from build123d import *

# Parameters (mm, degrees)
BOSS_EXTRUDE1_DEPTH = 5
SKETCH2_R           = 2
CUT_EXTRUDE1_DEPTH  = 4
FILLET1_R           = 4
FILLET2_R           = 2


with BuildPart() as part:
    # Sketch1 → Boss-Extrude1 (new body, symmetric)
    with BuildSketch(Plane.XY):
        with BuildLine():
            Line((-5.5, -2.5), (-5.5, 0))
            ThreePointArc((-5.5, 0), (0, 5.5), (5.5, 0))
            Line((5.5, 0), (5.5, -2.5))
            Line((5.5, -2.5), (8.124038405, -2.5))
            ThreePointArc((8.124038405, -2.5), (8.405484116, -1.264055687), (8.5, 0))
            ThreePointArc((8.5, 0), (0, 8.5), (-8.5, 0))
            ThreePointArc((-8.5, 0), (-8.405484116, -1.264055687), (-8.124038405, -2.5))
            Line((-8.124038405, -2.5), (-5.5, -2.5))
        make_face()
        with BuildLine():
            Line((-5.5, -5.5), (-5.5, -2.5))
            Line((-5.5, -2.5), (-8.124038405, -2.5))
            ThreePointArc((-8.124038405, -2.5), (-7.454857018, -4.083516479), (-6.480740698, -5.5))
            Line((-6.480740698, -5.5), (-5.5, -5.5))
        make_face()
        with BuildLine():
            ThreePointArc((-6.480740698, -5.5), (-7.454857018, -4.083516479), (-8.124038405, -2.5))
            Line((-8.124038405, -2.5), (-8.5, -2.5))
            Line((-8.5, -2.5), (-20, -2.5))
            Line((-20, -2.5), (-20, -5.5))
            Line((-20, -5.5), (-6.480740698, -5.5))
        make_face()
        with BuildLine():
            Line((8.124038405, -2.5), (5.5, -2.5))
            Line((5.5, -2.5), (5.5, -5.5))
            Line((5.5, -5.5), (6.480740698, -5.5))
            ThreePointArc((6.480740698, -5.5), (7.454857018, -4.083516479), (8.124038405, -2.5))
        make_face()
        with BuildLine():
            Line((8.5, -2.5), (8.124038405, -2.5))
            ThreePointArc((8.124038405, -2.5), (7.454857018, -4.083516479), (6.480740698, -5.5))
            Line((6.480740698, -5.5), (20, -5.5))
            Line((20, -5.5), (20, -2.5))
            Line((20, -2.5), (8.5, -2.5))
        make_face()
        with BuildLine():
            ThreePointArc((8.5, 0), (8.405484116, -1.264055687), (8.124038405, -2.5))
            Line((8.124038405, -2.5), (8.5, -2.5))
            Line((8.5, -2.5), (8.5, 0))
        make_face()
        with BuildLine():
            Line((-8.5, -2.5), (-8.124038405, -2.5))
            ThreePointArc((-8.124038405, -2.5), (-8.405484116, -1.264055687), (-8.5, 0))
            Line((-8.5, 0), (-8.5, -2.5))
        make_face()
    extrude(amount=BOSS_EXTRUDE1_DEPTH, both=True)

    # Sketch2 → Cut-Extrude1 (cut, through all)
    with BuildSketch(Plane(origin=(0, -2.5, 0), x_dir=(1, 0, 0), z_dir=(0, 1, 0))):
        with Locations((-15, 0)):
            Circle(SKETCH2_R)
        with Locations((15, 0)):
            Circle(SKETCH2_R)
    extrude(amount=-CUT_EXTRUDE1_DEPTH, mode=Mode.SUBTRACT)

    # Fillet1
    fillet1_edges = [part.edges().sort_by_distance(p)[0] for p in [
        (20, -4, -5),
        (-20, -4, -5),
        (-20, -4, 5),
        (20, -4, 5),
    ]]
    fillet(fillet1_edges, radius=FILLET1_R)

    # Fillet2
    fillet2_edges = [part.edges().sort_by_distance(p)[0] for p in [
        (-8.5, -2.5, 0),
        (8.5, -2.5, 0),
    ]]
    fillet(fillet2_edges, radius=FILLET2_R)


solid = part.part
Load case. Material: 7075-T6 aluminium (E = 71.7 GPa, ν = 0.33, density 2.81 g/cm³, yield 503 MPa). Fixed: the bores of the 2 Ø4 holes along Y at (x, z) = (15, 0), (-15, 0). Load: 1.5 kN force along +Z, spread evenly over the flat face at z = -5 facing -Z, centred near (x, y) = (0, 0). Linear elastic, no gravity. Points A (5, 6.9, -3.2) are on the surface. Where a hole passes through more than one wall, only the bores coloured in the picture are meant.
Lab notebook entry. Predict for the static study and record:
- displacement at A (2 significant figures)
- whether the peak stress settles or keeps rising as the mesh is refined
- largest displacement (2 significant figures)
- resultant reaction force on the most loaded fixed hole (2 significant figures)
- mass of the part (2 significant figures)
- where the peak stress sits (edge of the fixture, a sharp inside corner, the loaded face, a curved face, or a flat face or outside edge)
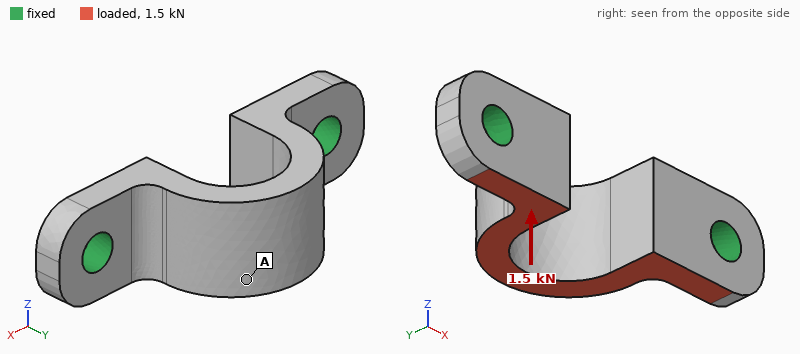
0.093 mm
keeps rising
0.11 mm
750 N
4.4 g
edge of the fixture
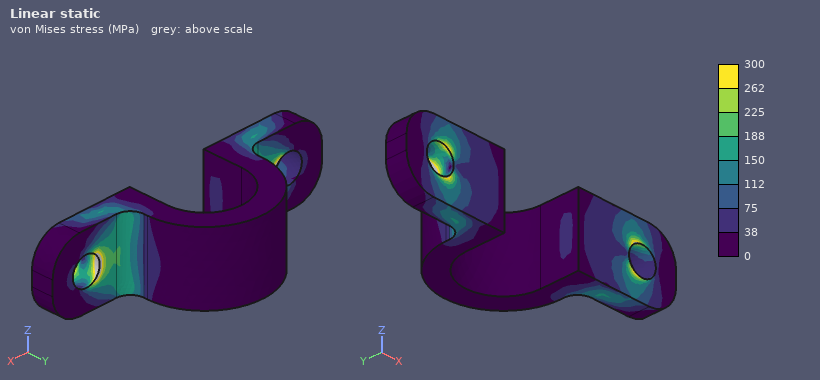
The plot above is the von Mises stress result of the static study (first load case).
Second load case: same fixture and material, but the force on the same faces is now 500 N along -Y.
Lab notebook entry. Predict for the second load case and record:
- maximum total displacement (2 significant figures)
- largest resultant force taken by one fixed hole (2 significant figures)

33 µm
260 N
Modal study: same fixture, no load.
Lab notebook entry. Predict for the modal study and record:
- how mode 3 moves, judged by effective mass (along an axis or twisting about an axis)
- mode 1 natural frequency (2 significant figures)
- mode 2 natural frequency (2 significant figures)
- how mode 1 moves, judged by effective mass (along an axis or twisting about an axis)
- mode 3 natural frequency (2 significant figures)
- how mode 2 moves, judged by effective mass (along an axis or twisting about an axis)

along Y
11 kHz
22 kHz
along Z
24 kHz
along X
